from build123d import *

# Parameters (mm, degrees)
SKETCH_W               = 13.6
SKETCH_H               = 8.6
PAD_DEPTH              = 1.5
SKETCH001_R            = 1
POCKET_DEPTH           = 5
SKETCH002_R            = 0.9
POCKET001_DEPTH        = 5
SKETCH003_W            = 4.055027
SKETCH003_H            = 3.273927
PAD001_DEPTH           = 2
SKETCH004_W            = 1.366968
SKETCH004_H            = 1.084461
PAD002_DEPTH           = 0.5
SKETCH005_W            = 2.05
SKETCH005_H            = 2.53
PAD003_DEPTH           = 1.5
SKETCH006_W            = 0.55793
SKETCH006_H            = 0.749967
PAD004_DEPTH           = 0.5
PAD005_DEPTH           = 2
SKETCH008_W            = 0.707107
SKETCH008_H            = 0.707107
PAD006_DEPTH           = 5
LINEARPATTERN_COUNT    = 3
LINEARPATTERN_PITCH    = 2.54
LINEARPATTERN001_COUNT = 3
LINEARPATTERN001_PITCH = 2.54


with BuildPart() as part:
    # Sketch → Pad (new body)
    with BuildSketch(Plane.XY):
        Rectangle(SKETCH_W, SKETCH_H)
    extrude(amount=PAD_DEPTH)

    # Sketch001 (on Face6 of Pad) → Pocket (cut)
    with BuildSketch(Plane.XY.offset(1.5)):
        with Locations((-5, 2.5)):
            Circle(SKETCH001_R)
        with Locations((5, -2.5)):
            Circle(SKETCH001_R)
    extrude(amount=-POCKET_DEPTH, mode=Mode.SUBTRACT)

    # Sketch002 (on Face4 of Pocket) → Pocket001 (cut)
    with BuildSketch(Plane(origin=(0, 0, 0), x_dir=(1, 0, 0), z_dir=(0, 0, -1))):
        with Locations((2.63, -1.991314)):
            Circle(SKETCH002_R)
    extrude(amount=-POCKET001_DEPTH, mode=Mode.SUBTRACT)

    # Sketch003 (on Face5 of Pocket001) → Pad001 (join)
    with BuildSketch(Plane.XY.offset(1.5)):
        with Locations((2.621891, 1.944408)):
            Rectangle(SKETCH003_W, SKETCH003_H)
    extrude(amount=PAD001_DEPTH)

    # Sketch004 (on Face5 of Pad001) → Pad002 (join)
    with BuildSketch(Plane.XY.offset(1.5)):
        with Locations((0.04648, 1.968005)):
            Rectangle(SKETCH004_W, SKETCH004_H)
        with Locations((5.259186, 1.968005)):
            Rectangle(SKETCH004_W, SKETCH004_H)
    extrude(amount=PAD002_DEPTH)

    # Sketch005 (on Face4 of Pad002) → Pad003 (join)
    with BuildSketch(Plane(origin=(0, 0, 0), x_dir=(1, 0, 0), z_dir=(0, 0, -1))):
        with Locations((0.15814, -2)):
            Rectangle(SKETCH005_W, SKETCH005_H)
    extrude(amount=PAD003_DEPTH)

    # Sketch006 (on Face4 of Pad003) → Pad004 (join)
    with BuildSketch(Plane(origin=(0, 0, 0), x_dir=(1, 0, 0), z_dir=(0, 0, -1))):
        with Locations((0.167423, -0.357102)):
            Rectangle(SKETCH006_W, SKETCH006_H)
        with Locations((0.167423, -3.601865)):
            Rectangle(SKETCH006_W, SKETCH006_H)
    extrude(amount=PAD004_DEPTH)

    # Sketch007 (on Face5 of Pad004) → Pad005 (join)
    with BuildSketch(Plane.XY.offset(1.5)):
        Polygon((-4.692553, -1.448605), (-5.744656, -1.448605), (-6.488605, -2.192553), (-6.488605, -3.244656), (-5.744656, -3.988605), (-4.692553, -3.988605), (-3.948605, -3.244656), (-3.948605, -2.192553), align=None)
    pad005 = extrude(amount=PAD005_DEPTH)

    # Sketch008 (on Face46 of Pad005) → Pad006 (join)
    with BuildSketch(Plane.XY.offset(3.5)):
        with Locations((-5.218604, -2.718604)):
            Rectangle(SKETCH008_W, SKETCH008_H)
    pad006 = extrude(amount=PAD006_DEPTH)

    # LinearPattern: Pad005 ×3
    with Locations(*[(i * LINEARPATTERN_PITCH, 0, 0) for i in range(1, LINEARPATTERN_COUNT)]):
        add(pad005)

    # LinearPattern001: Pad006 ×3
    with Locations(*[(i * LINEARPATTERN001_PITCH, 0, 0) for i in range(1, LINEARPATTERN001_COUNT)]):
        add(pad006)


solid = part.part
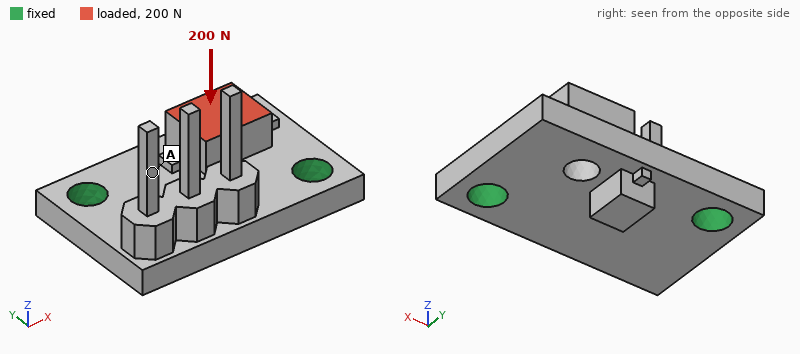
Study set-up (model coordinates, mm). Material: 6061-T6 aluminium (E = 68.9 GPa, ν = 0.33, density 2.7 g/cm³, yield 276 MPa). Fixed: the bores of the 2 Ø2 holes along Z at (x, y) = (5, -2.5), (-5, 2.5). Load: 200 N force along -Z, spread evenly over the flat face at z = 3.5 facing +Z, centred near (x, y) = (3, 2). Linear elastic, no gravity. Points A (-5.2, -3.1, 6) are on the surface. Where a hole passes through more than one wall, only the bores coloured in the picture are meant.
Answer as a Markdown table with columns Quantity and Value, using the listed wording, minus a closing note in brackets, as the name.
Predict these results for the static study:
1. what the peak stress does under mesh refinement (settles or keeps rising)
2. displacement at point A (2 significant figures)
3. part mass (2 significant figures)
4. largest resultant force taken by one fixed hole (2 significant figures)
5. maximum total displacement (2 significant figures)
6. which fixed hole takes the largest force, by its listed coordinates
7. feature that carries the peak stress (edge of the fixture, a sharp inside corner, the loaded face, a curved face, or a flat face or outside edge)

| Quantity | Value |
|---|---|
| what the peak stress does under mesh refinement | keeps rising |
| displacement at point A | 12 µm |
| part mass | 0.64 g |
| largest resultant force taken by one fixed hole | 130 N |
| maximum total displacement | 32 µm |
| which fixed hole takes the largest force, by its listed coordinates | (5, -2.5) |
| feature that carries the peak stress | edge of the fixture |
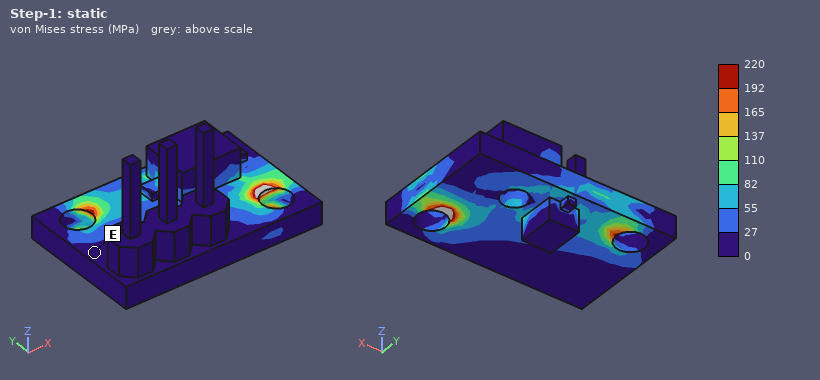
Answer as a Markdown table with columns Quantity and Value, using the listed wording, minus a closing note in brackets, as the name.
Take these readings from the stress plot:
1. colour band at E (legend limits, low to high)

| Quantity | Value |
|---|---|
| colour band at E | 0 to 27 MPa |
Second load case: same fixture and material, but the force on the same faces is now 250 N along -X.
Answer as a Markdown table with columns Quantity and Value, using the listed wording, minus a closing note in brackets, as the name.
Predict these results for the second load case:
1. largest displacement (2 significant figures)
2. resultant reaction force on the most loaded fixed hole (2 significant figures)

| Quantity | Value |
|---|---|
| largest displacement | 23 µm |
| resultant reaction force on the most loaded fixed hole | 150 N |
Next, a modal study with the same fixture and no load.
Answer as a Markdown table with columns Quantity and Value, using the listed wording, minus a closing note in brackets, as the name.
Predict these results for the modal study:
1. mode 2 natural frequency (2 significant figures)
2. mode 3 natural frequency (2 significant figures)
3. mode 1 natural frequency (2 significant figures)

| Quantity | Value |
|---|---|
| mode 2 natural frequency | 21 kHz |
| mode 3 natural frequency | 22 kHz |
| mode 1 natural frequency | 19 kHz |
